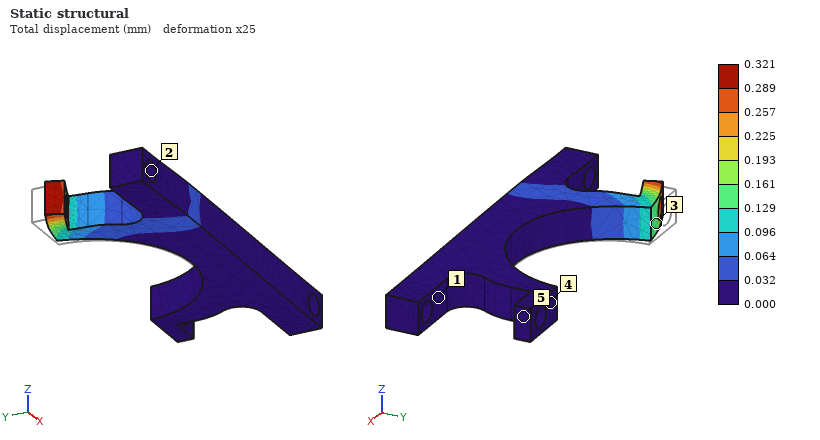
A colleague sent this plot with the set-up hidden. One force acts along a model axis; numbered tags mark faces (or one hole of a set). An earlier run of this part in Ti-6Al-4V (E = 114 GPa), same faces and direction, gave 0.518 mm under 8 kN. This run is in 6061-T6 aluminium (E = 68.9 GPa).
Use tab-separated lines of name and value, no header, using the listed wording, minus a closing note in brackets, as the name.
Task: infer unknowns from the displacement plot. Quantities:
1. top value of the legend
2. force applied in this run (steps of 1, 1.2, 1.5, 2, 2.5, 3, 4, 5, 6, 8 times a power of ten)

top value of the legend	0.321 mm
force applied in this run	3 kN
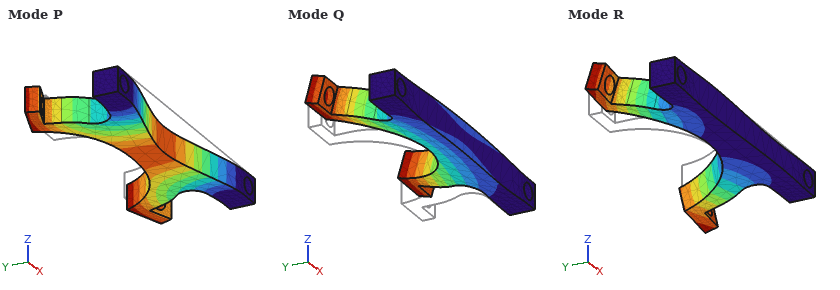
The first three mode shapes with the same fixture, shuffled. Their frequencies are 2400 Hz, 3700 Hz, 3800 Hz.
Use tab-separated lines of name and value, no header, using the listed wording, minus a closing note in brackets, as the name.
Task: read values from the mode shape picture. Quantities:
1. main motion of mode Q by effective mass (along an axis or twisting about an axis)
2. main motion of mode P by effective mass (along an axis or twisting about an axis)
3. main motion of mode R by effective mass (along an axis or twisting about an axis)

main motion of mode Q by effective mass	along Z
main motion of mode P by effective mass	along Y
main motion of mode R by effective mass	twisting about Y
